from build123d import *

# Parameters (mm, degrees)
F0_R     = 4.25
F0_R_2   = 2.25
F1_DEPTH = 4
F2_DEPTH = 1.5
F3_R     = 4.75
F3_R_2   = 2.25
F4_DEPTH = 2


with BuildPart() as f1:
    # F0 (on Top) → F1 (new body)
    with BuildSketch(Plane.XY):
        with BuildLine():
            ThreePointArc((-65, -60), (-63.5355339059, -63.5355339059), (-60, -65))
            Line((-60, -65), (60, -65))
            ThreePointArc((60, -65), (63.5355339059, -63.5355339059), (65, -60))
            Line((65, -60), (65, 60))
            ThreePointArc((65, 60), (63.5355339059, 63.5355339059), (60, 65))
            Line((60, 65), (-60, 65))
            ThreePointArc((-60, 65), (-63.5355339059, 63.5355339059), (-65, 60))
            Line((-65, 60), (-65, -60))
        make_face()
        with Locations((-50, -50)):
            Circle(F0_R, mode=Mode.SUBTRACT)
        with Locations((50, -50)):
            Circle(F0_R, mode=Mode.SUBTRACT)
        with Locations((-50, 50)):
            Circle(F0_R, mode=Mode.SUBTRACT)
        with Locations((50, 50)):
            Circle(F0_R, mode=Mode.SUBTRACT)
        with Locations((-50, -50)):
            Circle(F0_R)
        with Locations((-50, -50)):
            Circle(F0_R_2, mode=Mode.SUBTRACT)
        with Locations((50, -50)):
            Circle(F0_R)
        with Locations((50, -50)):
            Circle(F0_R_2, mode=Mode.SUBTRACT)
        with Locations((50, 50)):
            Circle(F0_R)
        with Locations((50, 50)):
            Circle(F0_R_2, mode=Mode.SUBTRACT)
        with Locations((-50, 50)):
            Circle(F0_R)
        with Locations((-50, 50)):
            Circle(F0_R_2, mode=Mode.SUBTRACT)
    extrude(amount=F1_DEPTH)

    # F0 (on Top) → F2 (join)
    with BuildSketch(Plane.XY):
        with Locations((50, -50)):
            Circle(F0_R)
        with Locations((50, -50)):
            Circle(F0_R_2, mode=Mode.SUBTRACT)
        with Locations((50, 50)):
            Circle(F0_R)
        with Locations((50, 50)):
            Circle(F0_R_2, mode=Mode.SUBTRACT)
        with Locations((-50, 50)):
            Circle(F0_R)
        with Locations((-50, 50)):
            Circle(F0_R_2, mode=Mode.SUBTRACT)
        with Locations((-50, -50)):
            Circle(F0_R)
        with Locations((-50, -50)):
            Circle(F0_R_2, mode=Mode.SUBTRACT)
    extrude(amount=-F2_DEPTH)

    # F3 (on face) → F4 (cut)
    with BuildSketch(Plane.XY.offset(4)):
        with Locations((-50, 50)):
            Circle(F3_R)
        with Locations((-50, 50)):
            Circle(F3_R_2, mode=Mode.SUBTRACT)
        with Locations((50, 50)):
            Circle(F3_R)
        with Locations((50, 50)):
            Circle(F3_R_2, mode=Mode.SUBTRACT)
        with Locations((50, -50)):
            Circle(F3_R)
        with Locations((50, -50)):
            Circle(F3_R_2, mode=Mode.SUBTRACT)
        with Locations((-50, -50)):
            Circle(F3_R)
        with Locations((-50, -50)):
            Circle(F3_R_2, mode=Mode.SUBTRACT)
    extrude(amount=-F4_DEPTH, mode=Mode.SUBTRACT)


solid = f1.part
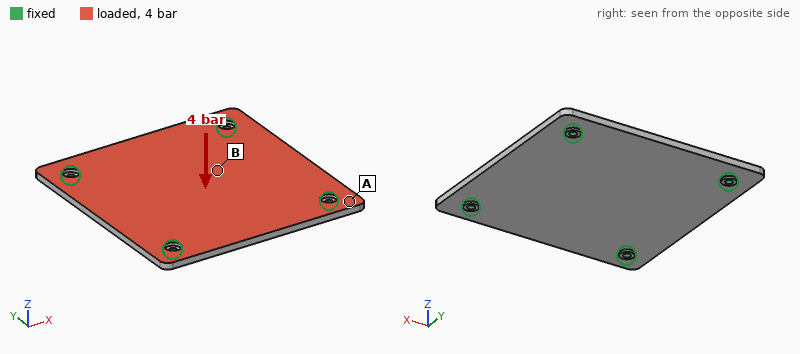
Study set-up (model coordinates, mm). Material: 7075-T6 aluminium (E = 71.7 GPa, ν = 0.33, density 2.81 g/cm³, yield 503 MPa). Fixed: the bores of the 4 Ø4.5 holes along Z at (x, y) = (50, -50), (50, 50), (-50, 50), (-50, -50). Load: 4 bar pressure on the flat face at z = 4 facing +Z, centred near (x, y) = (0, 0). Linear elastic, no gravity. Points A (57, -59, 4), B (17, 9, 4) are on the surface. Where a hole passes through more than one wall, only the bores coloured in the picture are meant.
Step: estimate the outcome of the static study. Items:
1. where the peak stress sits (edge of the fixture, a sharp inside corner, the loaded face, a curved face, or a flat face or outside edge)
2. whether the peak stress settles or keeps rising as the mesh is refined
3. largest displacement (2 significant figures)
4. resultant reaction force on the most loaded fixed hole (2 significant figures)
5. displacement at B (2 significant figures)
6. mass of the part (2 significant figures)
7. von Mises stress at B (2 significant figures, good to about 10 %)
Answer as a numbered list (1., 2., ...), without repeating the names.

1. edge of the fixture
2. keeps rising
3. 0.82 mm
4. 3.3 kN
5. 0.74 mm
6. 190 g
7. 84 MPa
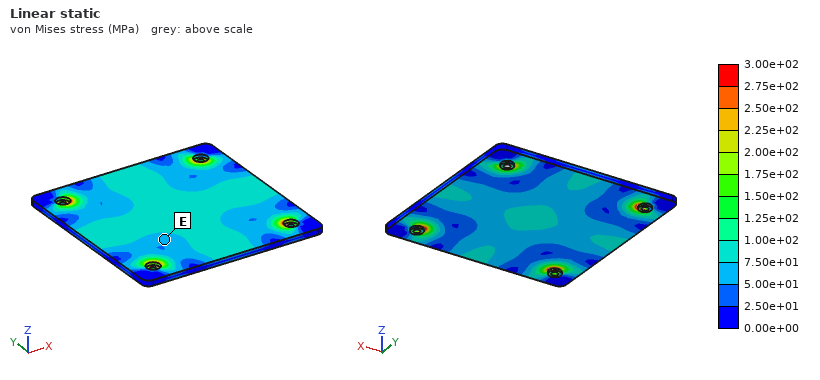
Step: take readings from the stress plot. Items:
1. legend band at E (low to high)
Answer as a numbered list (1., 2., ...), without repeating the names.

1. 5.00e+01 to 7.50e+01 MPa
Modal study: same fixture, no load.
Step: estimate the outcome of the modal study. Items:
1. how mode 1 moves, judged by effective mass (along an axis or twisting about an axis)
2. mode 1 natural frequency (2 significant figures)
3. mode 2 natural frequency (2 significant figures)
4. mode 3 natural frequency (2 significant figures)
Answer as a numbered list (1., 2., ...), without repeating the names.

1. along Z
2. 1300 Hz
3. 2000 Hz
4. 2000 Hz
